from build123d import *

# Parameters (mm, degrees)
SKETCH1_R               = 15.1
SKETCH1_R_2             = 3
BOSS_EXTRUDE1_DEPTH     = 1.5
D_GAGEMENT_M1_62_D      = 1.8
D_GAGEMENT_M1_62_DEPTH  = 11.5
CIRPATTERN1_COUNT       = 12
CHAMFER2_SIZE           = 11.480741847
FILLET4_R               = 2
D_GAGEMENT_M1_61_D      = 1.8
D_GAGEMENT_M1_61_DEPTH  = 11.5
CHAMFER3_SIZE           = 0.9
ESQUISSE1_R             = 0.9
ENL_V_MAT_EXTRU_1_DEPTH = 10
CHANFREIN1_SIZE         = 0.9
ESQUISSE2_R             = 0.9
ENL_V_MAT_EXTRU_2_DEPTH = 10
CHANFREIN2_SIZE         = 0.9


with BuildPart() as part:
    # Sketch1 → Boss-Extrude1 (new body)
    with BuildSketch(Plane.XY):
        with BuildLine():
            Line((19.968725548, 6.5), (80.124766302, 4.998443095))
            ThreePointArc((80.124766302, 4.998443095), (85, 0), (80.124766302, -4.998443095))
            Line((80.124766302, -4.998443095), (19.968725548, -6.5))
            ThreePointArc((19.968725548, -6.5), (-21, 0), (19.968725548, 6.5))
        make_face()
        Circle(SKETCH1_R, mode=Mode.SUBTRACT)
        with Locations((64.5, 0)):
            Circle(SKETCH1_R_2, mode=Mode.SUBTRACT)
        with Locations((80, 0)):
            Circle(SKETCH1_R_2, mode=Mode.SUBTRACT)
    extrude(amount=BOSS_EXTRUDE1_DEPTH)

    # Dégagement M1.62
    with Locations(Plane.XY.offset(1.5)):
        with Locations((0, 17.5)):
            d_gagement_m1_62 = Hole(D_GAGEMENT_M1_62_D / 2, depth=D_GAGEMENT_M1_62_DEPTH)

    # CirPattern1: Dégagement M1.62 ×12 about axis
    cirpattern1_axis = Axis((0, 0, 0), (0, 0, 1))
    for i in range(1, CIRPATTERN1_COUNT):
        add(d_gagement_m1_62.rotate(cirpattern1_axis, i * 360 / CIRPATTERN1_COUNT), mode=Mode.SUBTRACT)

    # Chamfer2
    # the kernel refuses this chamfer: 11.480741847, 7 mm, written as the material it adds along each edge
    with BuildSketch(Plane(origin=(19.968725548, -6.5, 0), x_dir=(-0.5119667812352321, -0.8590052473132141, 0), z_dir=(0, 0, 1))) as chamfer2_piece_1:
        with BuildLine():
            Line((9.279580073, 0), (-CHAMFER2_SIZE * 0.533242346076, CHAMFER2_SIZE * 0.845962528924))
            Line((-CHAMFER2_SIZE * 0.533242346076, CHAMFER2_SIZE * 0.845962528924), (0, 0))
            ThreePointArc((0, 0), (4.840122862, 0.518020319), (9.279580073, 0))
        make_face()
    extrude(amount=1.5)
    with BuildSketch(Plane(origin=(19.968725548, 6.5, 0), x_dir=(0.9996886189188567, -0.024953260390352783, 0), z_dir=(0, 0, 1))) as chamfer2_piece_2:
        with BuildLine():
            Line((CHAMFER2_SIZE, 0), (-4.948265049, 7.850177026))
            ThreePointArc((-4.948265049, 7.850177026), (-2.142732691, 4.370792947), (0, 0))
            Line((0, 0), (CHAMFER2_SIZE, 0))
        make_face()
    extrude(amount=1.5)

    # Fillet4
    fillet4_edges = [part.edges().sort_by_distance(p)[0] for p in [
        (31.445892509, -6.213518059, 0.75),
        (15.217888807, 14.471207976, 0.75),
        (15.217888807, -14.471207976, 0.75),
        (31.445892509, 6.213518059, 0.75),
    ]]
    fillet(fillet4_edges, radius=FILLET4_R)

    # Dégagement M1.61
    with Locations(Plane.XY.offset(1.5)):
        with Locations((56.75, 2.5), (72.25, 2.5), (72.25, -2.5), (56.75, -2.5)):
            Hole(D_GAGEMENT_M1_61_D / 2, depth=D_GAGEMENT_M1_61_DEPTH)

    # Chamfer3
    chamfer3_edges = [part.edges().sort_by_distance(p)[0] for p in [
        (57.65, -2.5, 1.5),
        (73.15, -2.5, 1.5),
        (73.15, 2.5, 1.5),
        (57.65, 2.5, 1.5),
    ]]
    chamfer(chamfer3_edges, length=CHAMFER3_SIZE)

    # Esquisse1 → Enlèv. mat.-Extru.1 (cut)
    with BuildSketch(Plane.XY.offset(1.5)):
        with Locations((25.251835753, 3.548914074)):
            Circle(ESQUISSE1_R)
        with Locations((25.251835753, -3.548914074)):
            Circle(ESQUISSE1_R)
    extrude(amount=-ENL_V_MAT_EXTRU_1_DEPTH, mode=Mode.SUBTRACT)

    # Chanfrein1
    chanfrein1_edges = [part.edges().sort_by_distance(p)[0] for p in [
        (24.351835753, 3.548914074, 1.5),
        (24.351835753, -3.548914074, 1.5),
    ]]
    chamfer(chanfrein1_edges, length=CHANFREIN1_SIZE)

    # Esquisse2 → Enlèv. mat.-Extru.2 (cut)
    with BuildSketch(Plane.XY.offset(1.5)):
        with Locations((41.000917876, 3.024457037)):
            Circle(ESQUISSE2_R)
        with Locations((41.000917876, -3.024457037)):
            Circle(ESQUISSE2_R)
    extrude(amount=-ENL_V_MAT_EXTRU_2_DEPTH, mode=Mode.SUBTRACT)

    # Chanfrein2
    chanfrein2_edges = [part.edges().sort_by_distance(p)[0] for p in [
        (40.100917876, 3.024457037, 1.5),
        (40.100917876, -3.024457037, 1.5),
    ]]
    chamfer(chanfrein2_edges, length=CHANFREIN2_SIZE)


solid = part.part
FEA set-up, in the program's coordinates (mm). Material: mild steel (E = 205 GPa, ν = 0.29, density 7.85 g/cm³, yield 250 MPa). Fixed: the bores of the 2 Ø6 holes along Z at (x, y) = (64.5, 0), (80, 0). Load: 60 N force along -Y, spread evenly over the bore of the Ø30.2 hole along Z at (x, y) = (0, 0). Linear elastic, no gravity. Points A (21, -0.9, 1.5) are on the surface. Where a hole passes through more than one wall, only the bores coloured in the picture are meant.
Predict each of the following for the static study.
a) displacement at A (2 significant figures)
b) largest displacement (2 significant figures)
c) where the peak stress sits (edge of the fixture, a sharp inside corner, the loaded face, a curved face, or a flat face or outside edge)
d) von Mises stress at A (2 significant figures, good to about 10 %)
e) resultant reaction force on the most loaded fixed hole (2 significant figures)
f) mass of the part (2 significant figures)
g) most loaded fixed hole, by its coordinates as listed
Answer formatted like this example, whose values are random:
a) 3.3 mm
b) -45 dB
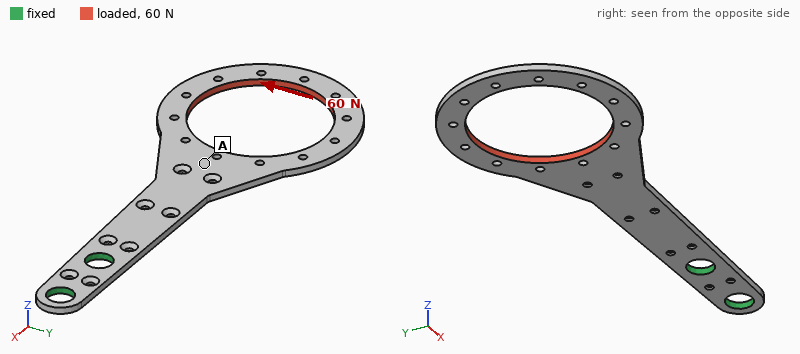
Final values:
a) 0.086 mm
b) 0.23 mm
c) a curved face
d) 15 MPa
e) 85 N
f) 16 g
g) (64.5, 0)
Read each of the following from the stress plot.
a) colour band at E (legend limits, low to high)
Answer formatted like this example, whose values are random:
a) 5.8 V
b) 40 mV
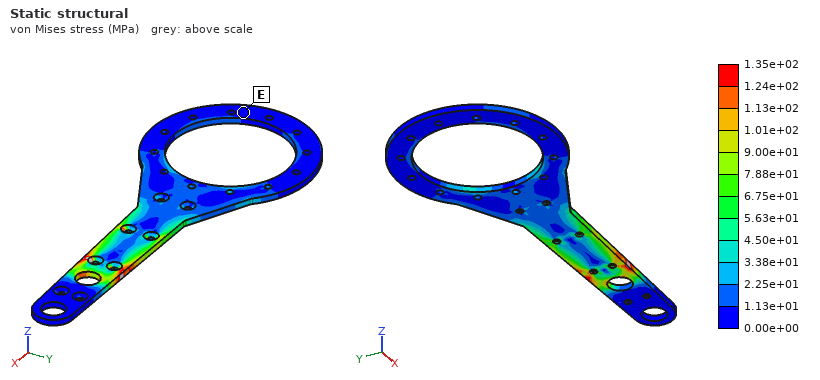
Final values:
a) 0.00e+00 to 1.13e+01 MPa
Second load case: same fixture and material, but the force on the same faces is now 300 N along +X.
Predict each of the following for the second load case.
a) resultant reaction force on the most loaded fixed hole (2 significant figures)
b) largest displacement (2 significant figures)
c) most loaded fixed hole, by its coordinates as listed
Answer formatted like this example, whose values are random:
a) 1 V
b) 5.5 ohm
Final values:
a) 290 N
b) 37 µm
c) (64.5, 0)
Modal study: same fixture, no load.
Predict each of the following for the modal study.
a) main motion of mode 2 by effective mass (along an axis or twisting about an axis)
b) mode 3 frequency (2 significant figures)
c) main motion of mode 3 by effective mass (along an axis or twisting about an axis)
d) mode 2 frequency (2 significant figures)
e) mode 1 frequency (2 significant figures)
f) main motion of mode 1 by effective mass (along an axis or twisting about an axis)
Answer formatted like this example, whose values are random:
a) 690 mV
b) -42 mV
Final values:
a) twisting about X
b) 910 Hz
c) along Z
d) 580 Hz
e) 150 Hz
f) along Z
